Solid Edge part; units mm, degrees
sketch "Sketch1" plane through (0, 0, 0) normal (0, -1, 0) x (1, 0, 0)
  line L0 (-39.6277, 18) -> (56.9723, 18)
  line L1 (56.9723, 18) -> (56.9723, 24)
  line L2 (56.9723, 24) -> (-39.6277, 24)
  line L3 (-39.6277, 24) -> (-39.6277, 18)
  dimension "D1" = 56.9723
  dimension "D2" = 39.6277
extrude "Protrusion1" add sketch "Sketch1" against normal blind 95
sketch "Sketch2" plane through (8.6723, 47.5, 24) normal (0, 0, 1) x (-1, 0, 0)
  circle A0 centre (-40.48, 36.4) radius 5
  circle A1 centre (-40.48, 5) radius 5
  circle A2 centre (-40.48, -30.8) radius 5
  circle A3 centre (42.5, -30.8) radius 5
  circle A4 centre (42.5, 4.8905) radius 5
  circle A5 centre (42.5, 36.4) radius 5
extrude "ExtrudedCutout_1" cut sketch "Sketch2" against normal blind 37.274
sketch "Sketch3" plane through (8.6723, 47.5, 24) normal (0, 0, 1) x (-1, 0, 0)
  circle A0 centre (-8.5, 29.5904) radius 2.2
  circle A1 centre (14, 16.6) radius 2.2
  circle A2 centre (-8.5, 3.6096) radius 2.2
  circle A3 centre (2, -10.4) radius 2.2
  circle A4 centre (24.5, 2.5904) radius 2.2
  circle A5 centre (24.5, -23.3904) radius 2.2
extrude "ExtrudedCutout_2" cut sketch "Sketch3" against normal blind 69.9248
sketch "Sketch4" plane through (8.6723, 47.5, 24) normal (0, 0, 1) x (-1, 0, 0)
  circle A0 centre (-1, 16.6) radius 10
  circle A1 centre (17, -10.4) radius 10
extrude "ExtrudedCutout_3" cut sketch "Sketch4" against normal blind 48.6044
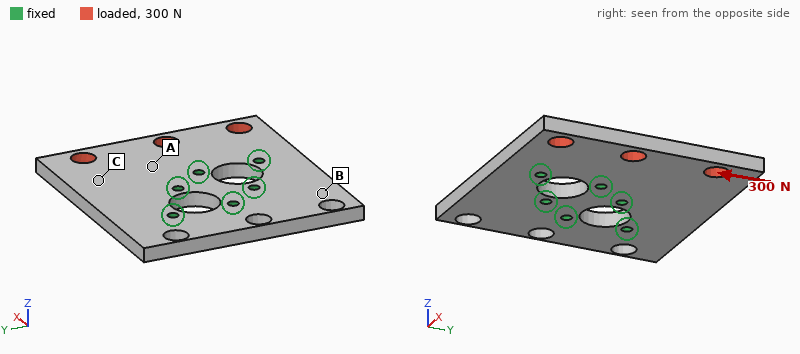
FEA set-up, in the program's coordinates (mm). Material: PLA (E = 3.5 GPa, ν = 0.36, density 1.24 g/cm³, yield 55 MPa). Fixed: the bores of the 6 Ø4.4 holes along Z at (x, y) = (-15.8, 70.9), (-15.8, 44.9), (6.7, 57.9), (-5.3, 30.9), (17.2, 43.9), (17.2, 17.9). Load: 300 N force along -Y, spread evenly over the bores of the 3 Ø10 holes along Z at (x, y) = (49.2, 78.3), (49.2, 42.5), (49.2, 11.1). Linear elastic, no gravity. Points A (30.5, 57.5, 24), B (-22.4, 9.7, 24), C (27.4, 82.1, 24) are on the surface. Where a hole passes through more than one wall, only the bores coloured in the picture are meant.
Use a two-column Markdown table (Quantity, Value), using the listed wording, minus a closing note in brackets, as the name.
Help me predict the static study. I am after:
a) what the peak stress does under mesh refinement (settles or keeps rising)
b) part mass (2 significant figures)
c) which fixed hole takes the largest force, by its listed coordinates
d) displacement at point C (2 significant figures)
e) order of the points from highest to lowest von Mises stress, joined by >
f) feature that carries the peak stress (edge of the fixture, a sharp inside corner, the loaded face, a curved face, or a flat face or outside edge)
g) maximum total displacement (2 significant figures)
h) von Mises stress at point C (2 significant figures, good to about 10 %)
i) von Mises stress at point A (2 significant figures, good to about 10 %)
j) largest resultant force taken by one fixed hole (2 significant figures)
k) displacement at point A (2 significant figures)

| Quantity | Value |
|---|---|
| what the peak stress does under mesh refinement | keeps rising |
| part mass | 59 g |
| which fixed hole takes the largest force, by its listed coordinates | (17.2, 17.9) |
| displacement at point C | 18 µm |
| order of the points from highest to lowest von Mises stress, joined by > | A > C > B |
| feature that carries the peak stress | edge of the fixture |
| maximum total displacement | 43 µm |
| von Mises stress at point C | 0.57 MPa |
| von Mises stress at point A | 1.1 MPa |
| largest resultant force taken by one fixed hole | 190 N |
| displacement at point A | 14 µm |
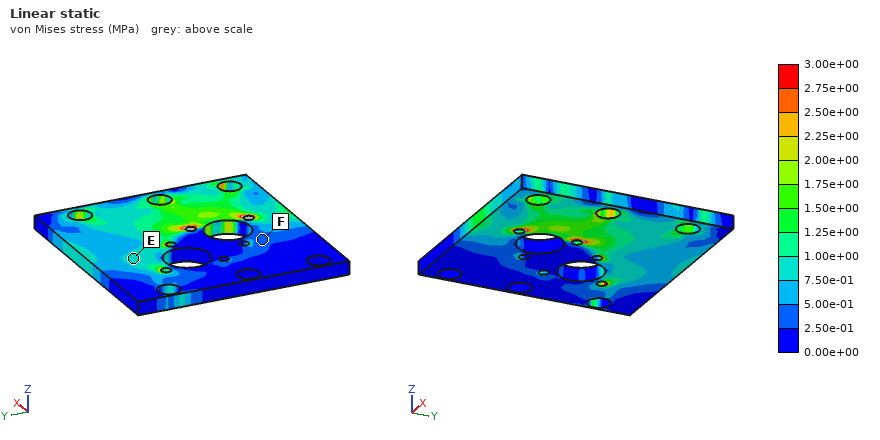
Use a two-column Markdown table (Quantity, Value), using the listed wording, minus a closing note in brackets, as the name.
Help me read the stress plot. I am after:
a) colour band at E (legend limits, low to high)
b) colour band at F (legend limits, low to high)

| Quantity | Value |
|---|---|
| colour band at E | 7.50e-01 to 1.00e+00 MPa |
| colour band at F | 2.50e-01 to 5.00e-01 MPa |
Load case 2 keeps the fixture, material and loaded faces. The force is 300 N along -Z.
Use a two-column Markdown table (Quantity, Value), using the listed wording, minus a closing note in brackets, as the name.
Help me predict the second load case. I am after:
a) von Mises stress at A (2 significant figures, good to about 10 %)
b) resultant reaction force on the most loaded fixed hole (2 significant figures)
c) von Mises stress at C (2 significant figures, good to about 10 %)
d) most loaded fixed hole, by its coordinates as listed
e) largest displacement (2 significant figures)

| Quantity | Value |
|---|---|
| von Mises stress at A | 9.4 MPa |
| resultant reaction force on the most loaded fixed hole | 220 N |
| von Mises stress at C | 7.1 MPa |
| most loaded fixed hole, by its coordinates as listed | (17.2, 43.9) |
| largest displacement | 1.5 mm |
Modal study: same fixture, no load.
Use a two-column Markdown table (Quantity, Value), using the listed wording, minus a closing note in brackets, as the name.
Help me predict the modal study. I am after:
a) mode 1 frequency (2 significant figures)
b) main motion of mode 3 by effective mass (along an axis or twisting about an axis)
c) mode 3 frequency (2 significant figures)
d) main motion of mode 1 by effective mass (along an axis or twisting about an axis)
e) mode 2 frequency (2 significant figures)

| Quantity | Value |
|---|---|
| mode 1 frequency | 690 Hz |
| main motion of mode 3 by effective mass | along Z |
| mode 3 frequency | 1300 Hz |
| main motion of mode 1 by effective mass | along Z |
| mode 2 frequency | 1100 Hz |
